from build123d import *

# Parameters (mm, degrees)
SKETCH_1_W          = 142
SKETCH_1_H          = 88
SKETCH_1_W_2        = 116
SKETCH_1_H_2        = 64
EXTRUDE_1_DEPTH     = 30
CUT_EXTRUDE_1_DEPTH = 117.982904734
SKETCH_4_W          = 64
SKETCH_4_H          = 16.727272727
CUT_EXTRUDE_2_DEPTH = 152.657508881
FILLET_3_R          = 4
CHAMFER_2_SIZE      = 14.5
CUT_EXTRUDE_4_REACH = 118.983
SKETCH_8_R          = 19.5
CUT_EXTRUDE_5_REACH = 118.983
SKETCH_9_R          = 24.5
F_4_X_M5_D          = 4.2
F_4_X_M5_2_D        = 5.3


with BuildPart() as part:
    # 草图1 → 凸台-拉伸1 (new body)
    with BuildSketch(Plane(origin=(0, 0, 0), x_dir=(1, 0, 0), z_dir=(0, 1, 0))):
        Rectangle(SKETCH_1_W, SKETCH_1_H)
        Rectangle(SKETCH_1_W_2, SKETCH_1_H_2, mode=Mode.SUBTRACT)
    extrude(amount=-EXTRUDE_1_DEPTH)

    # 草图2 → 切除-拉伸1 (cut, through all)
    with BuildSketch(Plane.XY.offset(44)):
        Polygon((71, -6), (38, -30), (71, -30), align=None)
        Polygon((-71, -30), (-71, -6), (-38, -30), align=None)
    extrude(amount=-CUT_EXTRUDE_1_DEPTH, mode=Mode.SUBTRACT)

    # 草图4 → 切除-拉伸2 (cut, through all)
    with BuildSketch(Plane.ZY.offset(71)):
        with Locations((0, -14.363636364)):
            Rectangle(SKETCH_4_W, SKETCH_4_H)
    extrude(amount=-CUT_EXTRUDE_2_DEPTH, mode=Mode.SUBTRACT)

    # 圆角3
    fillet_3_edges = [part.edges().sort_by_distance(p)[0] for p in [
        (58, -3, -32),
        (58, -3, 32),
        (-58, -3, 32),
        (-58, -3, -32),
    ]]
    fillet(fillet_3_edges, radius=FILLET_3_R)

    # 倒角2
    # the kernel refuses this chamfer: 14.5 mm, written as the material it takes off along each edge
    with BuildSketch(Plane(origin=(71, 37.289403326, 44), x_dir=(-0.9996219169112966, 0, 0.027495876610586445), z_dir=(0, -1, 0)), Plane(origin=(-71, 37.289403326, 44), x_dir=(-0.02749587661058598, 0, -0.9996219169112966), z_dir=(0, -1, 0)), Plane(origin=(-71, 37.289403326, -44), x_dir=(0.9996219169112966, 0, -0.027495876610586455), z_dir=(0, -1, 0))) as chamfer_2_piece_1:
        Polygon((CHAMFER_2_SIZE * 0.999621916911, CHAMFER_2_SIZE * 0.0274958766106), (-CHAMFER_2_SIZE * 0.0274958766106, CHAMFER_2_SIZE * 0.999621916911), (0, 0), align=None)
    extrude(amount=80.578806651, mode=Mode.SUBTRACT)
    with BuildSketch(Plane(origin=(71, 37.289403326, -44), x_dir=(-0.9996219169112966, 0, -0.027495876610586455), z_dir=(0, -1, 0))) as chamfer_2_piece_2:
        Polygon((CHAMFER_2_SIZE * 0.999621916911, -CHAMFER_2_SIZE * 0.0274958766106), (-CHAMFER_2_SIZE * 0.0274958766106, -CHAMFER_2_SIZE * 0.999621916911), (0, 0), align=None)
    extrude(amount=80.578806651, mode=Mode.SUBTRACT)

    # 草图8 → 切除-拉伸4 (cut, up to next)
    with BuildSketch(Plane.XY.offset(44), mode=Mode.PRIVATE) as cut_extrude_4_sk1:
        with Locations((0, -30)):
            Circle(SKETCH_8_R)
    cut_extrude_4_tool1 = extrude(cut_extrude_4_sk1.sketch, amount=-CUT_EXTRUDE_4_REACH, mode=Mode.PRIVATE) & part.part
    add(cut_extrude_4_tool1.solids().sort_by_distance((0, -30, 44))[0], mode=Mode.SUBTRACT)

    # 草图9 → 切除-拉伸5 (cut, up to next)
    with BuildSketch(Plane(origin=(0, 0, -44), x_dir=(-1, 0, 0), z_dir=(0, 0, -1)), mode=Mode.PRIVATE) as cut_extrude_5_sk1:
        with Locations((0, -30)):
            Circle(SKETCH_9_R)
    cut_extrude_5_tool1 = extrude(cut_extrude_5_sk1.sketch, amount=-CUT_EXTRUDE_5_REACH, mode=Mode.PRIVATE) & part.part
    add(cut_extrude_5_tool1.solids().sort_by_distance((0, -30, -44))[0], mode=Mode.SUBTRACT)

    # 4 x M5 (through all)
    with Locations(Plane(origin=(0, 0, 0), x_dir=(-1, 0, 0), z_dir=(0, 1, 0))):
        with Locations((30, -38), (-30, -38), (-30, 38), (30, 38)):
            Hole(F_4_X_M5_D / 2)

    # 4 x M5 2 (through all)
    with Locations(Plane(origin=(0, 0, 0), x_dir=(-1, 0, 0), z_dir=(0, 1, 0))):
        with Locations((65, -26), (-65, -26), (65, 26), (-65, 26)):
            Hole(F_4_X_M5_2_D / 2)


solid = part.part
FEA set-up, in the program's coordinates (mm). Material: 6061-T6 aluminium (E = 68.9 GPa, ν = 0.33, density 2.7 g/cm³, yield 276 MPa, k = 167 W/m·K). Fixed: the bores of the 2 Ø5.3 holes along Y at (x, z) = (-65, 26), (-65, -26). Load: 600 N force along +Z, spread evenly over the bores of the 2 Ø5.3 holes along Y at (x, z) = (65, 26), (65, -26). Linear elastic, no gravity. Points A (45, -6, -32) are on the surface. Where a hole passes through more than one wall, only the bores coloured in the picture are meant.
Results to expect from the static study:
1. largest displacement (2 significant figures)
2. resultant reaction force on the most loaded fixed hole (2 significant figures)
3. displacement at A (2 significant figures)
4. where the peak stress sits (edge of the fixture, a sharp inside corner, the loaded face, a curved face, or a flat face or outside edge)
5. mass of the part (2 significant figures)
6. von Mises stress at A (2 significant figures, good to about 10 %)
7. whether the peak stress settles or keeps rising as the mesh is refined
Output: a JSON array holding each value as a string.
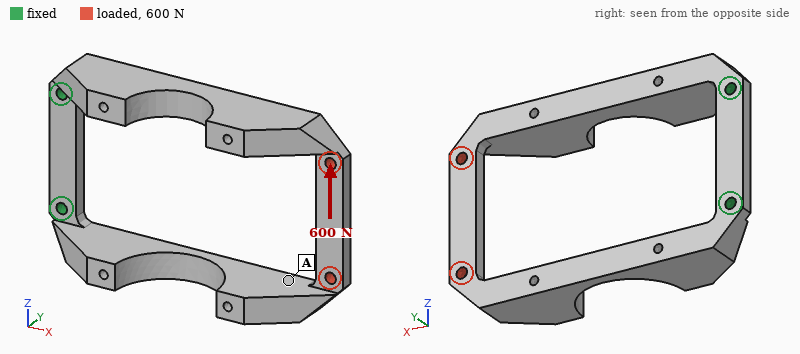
["1.2 mm", "820 N", "1.0 mm", "a sharp inside corner", "190 g", "31 MPa", "keeps rising"]
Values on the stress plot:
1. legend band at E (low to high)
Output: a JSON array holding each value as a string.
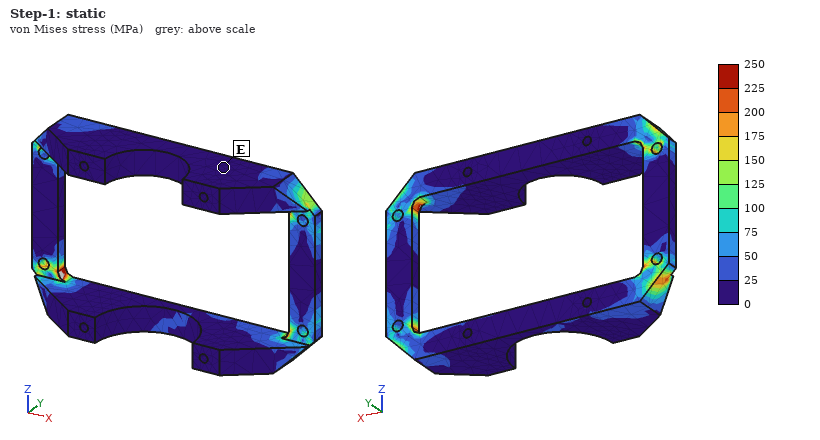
["0 to 25 MPa"]
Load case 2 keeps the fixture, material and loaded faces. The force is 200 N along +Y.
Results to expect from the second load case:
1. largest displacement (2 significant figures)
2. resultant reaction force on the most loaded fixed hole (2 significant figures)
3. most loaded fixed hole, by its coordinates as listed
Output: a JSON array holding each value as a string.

["1.3 mm", "120 N", "(-65, 26)"]
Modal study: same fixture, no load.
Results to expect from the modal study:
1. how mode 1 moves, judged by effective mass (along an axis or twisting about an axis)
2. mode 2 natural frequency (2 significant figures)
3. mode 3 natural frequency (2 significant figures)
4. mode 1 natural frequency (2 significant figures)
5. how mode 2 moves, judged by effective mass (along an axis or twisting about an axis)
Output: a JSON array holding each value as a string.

["along Y", "410 Hz", "570 Hz", "270 Hz", "along Z"]
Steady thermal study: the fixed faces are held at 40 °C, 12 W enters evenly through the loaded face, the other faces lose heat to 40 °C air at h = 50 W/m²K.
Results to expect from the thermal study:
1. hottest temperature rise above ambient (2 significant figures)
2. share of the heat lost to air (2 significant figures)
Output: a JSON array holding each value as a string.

["19 K", "70 %"]
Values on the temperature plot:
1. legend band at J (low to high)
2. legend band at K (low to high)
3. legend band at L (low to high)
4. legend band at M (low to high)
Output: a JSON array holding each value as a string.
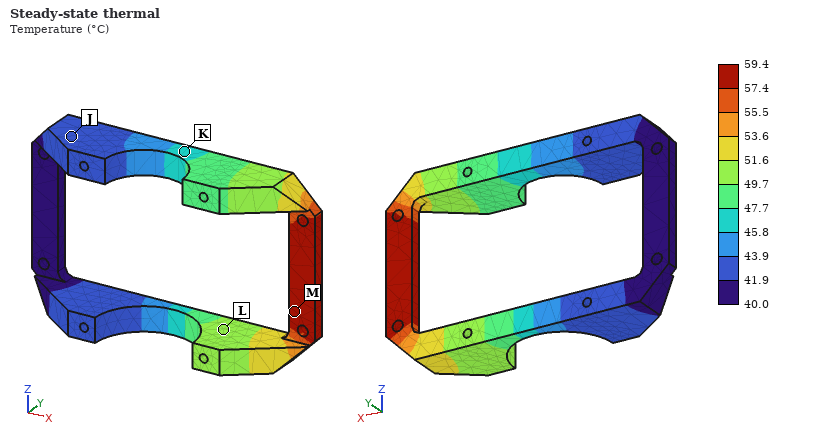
["41.9 to 43.9 °C", "45.8 to 47.7 °C", "49.7 to 51.6 °C", "57.4 to 59.4 °C"]
